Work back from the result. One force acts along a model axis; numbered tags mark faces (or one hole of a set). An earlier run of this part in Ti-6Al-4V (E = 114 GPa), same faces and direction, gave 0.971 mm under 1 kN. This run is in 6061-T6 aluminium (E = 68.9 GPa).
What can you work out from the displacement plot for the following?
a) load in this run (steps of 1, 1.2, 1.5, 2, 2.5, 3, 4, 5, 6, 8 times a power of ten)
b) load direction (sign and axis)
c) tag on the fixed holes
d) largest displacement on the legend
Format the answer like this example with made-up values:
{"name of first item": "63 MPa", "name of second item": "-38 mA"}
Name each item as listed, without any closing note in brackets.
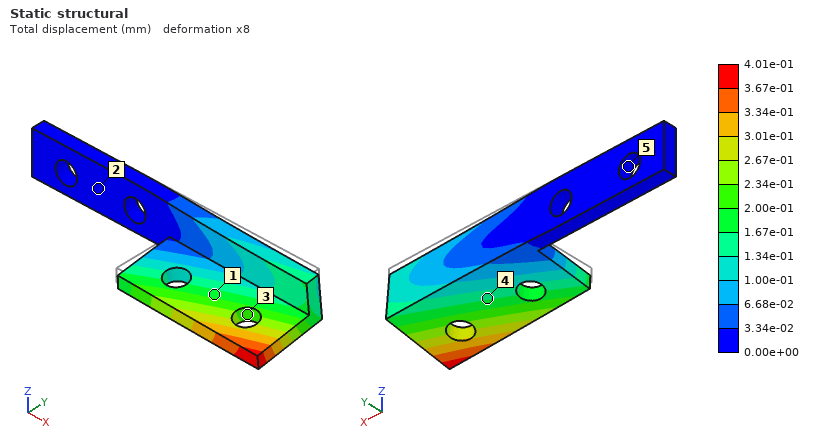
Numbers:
{"load in this run": "250 N", "load direction": "-Z", "tag on the fixed holes": "5", "largest displacement on the legend": "4.01e-01 mm"}
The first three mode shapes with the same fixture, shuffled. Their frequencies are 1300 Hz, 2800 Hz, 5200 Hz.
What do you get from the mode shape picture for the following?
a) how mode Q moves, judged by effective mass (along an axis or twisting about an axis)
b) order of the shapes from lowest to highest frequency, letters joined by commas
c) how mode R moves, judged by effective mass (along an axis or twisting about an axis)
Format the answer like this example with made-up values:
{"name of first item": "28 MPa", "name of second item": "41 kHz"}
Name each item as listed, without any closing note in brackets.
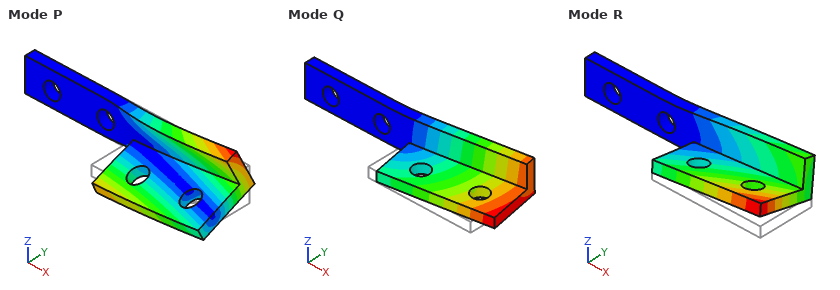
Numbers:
{"how mode Q moves, judged by effective mass": "along Y", "order of the shapes from lowest to highest frequency, letters joined by commas": "Q, R, P", "how mode R moves, judged by effective mass": "along Z"}
